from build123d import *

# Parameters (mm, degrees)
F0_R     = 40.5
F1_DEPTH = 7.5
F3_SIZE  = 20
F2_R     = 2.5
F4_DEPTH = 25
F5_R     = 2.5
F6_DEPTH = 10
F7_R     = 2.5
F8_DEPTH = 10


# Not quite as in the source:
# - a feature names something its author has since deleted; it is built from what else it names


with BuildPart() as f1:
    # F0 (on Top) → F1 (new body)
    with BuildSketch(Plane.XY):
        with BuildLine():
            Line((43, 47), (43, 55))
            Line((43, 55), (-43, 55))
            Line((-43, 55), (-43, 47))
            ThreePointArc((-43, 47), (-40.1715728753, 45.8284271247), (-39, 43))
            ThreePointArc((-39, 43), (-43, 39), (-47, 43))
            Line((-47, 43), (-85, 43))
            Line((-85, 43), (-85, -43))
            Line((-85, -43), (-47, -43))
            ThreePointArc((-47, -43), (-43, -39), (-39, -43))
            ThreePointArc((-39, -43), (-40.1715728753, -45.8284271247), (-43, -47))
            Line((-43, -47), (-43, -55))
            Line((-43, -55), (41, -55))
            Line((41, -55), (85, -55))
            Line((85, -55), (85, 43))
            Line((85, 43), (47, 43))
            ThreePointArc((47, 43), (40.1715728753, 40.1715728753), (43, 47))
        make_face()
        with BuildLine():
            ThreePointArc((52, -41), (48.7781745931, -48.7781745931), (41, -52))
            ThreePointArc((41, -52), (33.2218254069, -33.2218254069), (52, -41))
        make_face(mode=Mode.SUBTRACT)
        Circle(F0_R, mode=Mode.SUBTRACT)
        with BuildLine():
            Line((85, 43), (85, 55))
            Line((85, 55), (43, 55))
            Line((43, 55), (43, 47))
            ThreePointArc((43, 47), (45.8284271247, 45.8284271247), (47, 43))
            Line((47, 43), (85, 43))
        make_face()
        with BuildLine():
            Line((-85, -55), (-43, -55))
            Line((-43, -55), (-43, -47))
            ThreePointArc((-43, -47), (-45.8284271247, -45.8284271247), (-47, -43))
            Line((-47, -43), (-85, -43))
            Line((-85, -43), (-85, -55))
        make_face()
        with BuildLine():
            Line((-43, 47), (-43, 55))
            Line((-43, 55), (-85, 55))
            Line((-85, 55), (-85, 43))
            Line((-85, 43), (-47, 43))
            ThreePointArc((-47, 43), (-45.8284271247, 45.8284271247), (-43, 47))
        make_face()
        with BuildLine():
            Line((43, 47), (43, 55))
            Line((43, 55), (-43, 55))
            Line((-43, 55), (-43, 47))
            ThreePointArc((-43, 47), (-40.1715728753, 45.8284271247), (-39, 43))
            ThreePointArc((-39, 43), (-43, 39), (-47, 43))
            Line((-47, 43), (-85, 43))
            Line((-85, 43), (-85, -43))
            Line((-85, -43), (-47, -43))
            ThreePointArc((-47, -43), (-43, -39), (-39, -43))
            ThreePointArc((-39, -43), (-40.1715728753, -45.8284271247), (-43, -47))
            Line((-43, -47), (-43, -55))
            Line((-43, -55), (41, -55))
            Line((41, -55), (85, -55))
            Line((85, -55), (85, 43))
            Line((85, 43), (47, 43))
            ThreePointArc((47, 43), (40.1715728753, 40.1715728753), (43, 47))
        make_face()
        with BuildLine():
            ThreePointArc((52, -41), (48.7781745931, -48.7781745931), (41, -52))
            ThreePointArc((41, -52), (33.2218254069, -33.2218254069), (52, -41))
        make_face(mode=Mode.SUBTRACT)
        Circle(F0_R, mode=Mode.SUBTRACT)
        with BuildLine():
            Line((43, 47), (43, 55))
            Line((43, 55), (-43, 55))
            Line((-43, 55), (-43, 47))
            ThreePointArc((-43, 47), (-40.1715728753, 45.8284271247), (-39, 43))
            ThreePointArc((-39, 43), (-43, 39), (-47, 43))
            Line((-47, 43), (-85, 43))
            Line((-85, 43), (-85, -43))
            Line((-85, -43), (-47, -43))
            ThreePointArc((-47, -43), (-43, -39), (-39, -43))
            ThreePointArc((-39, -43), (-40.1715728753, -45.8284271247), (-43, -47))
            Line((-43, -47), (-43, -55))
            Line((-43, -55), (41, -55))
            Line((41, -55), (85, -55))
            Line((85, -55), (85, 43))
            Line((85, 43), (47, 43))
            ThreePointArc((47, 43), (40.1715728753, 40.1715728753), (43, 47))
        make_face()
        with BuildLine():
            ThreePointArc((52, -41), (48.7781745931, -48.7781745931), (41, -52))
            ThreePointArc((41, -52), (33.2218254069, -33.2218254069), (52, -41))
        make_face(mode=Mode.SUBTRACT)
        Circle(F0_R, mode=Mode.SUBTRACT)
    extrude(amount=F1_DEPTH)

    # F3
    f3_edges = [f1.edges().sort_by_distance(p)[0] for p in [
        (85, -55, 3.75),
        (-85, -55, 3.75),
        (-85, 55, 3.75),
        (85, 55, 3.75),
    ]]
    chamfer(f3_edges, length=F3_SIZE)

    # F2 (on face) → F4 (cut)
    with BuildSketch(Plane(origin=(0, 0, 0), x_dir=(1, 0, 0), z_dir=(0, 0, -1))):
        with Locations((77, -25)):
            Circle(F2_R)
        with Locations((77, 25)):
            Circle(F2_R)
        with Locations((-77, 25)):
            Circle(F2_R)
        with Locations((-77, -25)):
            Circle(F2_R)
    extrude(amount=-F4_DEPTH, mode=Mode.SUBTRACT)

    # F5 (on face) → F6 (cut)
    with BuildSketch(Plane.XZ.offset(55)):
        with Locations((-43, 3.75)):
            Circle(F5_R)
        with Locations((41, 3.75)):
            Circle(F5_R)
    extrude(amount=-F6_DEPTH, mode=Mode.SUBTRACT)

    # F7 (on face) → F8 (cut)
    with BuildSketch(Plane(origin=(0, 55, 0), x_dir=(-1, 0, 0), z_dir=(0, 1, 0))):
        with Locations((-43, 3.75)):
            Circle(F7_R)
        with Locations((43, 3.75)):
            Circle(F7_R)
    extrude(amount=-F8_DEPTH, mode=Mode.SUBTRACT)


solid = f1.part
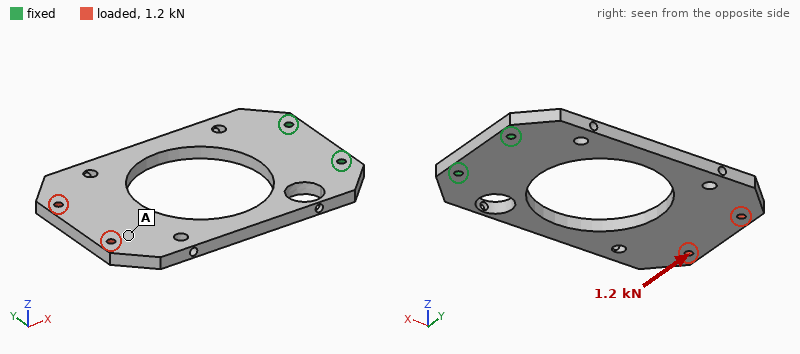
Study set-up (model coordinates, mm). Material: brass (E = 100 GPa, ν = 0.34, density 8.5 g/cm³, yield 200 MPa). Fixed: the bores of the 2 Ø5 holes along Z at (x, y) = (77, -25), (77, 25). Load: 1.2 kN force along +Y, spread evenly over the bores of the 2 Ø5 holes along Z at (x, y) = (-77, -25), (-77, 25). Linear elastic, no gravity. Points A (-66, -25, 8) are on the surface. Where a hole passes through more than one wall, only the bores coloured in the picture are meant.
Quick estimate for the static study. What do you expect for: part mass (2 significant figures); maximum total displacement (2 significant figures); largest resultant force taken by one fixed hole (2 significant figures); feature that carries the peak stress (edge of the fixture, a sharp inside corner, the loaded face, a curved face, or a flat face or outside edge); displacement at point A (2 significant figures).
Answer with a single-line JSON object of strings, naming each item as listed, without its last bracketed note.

{"part mass": "770 g", "maximum total displacement": "0.16 mm", "largest resultant force taken by one fixed hole": "3.5 kN", "feature that carries the peak stress": "a curved face", "displacement at point A": "0.14 mm"}
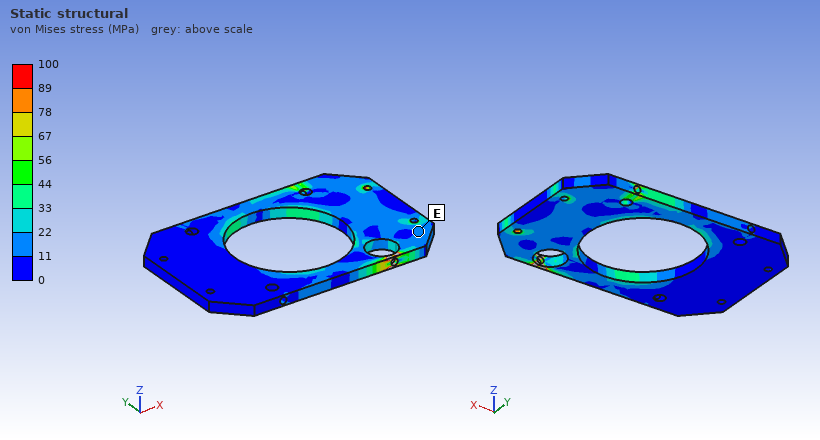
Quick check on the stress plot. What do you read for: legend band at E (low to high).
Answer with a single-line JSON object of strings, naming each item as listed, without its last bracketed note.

{"legend band at E": "11 to 22 MPa"}
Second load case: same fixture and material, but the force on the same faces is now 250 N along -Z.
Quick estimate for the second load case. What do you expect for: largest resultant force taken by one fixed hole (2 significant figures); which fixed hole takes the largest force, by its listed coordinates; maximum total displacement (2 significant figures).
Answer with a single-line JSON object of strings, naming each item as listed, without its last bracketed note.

{"largest resultant force taken by one fixed hole": "130 N", "which fixed hole takes the largest force, by its listed coordinates": "(77, 25)", "maximum total displacement": "2.1 mm"}
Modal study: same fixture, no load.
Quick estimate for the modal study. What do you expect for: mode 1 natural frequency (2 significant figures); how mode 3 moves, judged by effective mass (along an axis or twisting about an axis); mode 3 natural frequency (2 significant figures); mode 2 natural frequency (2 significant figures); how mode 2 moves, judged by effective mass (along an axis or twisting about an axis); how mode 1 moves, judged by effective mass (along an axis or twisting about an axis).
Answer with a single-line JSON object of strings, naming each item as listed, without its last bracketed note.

{"mode 1 natural frequency": "120 Hz", "how mode 3 moves, judged by effective mass": "along Y", "mode 3 natural frequency": "790 Hz", "mode 2 natural frequency": "390 Hz", "how mode 2 moves, judged by effective mass": "twisting about X", "how mode 1 moves, judged by effective mass": "along Z"}
